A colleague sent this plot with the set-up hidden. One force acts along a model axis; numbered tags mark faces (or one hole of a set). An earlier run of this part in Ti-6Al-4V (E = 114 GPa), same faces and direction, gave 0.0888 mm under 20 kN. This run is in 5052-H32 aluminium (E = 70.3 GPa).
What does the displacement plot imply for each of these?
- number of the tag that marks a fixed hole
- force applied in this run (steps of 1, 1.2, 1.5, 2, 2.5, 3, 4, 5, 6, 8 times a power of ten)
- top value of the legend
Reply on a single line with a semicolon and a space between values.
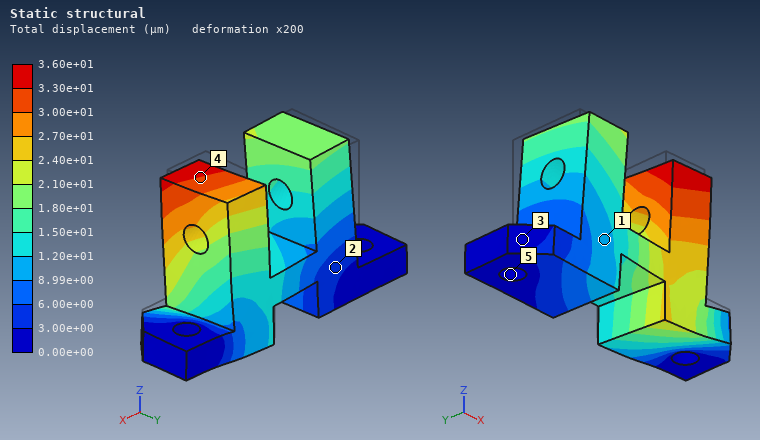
5; 5 kN; 3.60e+01 µm
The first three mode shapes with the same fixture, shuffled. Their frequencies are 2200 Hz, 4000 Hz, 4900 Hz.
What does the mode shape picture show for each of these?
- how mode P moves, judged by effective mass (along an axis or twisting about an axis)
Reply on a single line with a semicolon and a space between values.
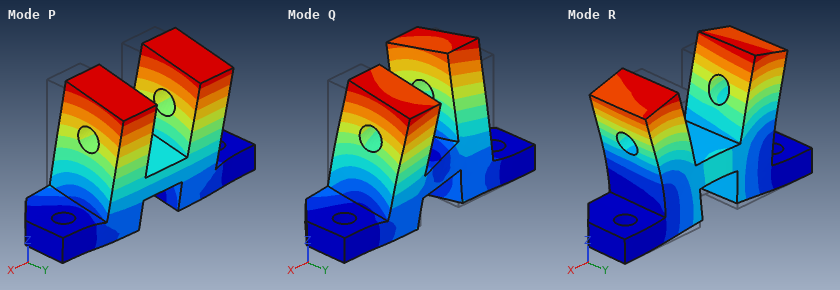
along Y
